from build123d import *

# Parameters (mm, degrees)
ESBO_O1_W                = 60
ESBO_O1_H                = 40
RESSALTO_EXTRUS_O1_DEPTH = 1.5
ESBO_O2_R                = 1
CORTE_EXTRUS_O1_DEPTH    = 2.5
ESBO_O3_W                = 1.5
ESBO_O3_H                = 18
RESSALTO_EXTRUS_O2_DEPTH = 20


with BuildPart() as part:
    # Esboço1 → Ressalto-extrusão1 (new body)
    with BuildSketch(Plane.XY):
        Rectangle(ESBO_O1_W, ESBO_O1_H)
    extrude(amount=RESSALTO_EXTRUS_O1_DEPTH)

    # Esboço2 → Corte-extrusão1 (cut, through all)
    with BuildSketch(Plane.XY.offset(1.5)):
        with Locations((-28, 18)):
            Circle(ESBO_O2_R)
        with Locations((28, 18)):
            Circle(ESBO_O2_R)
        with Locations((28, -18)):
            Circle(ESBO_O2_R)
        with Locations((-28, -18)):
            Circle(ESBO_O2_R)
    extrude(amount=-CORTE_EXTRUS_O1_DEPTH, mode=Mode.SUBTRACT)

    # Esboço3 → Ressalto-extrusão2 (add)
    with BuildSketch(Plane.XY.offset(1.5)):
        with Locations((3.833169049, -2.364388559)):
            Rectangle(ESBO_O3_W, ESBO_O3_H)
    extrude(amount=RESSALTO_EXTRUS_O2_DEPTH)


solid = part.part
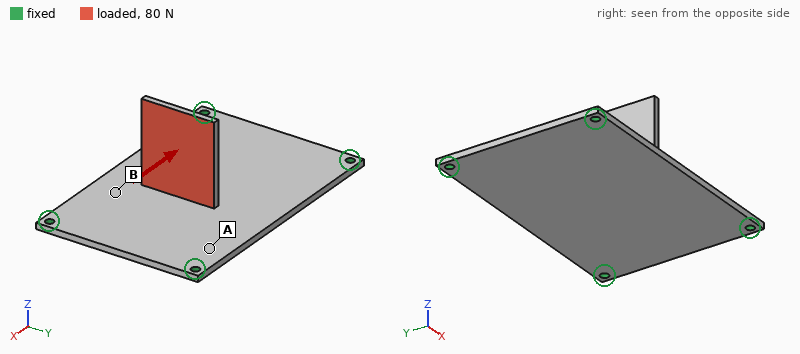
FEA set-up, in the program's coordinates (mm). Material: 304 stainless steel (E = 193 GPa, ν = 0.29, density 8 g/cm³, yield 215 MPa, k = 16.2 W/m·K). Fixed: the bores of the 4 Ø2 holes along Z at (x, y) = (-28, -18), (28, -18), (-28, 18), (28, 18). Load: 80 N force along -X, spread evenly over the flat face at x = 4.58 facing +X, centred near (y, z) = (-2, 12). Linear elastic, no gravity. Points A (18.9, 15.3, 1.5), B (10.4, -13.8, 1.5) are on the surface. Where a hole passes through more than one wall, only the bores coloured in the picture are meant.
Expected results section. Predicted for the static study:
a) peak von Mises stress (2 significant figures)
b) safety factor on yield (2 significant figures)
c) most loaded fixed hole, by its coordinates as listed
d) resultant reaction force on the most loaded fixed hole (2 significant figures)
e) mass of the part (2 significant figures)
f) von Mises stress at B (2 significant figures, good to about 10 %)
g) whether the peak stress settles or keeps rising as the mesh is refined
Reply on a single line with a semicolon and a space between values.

120 MPa; 1.8; (28, -18); 27 N; 33 g; 17 MPa; settles
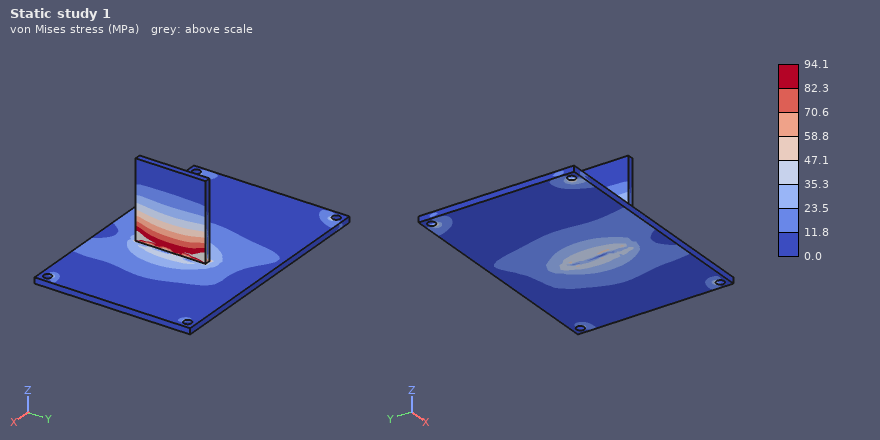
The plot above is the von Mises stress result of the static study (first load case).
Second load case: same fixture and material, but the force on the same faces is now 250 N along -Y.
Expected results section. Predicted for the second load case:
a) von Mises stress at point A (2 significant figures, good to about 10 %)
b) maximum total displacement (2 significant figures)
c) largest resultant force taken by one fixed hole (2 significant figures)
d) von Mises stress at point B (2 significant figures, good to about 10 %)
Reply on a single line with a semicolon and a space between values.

38 MPa; 0.13 mm; 100 N; 47 MPa
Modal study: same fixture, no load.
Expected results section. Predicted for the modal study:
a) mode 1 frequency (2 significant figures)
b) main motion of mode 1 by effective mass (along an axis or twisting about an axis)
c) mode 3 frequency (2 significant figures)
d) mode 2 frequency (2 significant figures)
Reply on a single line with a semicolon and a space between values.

1600 Hz; along Z; 2600 Hz; 2400 Hz
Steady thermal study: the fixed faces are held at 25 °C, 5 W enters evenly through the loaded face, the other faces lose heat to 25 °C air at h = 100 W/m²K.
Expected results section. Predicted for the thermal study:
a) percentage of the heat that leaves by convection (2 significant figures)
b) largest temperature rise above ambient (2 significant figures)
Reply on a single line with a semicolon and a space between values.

96 %; 70 K
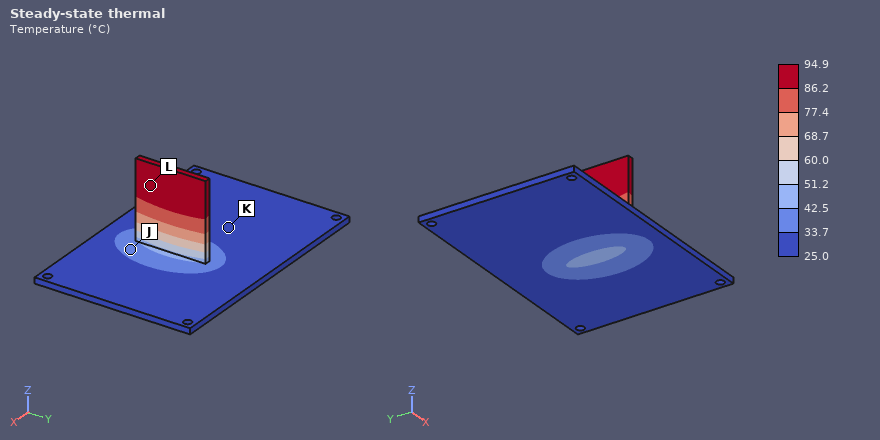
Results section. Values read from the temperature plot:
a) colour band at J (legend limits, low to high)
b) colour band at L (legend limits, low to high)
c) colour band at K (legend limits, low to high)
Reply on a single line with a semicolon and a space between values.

33.7 to 42.5 °C; 86.2 to 94.9 °C; 25.0 to 33.7 °C
